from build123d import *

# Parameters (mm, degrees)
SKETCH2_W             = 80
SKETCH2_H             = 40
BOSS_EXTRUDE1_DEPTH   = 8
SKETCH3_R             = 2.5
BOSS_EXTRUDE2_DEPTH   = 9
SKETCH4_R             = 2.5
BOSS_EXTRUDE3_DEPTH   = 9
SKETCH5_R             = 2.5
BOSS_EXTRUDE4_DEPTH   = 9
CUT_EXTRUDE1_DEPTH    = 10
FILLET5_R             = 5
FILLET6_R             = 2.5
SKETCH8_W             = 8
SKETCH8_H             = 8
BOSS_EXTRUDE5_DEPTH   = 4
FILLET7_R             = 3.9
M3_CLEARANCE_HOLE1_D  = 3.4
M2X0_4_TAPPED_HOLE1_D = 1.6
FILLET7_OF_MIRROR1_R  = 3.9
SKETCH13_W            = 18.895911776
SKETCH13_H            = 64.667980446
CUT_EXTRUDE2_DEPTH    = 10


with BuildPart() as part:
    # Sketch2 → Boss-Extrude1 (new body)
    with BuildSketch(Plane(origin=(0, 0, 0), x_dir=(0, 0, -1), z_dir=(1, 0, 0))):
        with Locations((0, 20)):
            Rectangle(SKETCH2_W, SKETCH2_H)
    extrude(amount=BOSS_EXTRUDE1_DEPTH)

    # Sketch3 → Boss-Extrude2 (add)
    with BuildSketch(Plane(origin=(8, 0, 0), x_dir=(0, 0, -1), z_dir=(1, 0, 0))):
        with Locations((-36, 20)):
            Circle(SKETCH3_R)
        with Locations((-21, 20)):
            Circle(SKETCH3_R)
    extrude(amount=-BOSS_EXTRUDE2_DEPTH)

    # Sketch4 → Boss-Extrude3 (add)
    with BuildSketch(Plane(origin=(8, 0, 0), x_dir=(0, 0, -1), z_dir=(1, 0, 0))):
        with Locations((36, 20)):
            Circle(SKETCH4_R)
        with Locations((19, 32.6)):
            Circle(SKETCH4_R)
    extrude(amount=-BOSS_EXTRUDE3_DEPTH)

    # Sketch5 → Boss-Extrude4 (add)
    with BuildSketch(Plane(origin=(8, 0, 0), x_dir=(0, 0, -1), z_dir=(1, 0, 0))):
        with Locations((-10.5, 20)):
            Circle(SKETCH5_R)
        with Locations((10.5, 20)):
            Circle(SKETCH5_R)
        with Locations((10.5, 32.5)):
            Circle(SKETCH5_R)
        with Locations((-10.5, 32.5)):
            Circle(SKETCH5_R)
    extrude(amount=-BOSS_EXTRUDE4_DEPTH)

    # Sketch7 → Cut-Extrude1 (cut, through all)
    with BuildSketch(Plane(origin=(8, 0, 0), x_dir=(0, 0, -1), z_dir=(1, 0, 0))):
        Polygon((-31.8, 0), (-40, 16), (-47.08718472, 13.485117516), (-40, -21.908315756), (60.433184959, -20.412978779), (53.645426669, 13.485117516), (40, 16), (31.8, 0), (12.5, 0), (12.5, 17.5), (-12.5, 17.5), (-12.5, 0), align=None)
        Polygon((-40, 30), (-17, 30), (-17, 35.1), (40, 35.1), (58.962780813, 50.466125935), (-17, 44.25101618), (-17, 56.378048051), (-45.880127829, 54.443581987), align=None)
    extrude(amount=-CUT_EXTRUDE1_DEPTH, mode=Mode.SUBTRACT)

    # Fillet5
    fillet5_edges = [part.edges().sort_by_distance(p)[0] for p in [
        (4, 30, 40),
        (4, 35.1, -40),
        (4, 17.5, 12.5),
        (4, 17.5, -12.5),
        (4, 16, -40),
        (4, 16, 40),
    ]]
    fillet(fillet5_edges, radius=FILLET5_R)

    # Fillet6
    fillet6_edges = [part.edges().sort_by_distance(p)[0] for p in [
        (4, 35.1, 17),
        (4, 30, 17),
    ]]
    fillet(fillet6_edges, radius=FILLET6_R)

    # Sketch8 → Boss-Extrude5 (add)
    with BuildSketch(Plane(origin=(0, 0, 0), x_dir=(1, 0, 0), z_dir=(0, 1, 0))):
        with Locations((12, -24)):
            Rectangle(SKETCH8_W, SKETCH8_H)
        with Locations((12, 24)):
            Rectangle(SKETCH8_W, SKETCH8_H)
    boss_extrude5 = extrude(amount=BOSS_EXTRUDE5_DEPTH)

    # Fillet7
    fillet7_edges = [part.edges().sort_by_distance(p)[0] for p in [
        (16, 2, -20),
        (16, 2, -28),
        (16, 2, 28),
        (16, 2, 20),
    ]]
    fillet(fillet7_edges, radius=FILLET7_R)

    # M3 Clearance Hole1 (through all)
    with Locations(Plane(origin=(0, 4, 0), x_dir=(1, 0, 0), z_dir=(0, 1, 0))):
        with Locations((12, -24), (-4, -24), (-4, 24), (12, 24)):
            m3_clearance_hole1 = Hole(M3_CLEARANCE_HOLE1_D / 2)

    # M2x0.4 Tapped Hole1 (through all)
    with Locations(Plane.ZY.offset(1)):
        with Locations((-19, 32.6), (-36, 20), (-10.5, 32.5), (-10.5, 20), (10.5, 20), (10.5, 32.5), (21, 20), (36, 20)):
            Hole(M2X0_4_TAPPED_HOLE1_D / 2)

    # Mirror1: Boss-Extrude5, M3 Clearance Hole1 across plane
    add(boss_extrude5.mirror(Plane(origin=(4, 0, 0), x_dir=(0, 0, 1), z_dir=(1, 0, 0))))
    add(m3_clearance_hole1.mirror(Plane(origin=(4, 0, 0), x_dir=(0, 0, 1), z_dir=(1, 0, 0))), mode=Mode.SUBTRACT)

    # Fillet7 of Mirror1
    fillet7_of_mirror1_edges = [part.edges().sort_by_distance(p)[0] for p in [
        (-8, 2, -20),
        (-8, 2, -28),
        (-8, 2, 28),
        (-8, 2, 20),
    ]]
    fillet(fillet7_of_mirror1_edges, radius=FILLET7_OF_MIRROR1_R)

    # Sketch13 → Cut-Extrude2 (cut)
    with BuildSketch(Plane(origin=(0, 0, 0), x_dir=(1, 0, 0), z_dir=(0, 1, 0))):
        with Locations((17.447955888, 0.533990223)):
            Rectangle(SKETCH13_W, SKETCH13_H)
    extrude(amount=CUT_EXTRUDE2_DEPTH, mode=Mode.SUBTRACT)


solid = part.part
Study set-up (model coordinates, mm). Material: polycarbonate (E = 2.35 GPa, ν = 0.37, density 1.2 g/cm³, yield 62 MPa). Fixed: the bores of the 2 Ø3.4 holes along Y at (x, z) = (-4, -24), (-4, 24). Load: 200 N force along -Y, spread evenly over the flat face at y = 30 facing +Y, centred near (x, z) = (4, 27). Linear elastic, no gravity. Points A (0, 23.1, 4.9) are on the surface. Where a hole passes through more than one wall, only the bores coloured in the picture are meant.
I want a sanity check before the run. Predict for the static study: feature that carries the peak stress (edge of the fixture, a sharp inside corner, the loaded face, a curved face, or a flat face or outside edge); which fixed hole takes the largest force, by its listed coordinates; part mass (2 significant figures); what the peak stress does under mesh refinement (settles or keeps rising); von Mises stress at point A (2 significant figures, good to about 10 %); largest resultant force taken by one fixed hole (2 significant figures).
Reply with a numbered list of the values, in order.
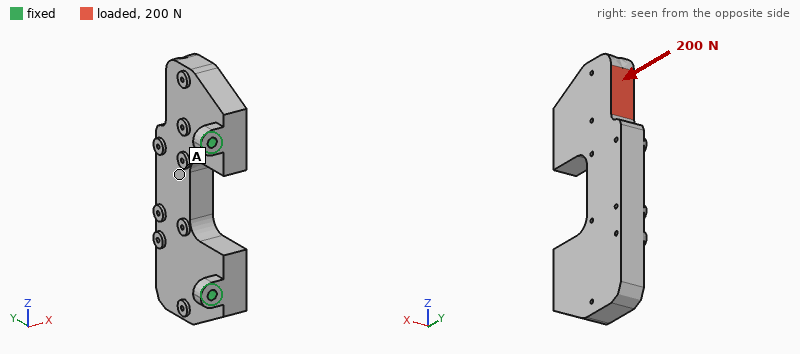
1. edge of the fixture
2. (-4, 24)
3. 21 g
4. keeps rising
5. 2.0 MPa
6. 210 N
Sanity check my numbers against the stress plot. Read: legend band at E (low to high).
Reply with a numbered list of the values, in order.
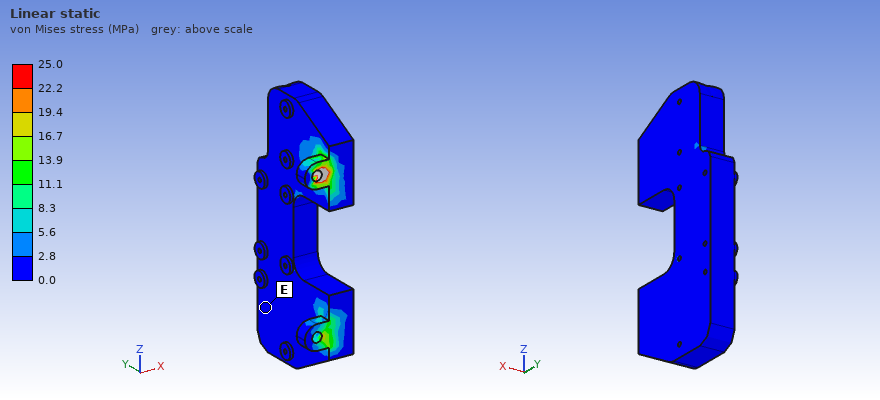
1. 0.0 to 2.8 MPa
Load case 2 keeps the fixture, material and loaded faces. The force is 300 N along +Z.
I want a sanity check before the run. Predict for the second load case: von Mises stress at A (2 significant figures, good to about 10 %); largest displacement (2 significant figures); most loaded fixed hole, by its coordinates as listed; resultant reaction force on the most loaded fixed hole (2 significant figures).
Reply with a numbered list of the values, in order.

1. 4.2 MPa
2. 0.34 mm
3. (-4, -24)
4. 240 N
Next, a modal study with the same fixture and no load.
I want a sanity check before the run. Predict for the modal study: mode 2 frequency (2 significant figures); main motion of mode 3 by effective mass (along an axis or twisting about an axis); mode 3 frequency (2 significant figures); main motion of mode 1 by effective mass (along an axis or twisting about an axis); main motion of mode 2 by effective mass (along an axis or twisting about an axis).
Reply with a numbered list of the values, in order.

1. 950 Hz
2. along Z
3. 1600 Hz
4. along X
5. twisting about Y
